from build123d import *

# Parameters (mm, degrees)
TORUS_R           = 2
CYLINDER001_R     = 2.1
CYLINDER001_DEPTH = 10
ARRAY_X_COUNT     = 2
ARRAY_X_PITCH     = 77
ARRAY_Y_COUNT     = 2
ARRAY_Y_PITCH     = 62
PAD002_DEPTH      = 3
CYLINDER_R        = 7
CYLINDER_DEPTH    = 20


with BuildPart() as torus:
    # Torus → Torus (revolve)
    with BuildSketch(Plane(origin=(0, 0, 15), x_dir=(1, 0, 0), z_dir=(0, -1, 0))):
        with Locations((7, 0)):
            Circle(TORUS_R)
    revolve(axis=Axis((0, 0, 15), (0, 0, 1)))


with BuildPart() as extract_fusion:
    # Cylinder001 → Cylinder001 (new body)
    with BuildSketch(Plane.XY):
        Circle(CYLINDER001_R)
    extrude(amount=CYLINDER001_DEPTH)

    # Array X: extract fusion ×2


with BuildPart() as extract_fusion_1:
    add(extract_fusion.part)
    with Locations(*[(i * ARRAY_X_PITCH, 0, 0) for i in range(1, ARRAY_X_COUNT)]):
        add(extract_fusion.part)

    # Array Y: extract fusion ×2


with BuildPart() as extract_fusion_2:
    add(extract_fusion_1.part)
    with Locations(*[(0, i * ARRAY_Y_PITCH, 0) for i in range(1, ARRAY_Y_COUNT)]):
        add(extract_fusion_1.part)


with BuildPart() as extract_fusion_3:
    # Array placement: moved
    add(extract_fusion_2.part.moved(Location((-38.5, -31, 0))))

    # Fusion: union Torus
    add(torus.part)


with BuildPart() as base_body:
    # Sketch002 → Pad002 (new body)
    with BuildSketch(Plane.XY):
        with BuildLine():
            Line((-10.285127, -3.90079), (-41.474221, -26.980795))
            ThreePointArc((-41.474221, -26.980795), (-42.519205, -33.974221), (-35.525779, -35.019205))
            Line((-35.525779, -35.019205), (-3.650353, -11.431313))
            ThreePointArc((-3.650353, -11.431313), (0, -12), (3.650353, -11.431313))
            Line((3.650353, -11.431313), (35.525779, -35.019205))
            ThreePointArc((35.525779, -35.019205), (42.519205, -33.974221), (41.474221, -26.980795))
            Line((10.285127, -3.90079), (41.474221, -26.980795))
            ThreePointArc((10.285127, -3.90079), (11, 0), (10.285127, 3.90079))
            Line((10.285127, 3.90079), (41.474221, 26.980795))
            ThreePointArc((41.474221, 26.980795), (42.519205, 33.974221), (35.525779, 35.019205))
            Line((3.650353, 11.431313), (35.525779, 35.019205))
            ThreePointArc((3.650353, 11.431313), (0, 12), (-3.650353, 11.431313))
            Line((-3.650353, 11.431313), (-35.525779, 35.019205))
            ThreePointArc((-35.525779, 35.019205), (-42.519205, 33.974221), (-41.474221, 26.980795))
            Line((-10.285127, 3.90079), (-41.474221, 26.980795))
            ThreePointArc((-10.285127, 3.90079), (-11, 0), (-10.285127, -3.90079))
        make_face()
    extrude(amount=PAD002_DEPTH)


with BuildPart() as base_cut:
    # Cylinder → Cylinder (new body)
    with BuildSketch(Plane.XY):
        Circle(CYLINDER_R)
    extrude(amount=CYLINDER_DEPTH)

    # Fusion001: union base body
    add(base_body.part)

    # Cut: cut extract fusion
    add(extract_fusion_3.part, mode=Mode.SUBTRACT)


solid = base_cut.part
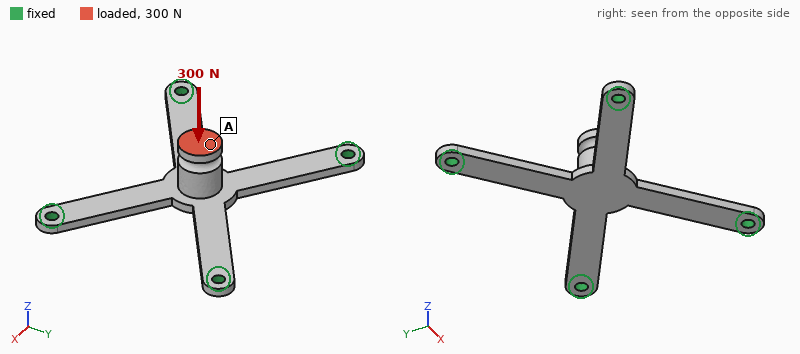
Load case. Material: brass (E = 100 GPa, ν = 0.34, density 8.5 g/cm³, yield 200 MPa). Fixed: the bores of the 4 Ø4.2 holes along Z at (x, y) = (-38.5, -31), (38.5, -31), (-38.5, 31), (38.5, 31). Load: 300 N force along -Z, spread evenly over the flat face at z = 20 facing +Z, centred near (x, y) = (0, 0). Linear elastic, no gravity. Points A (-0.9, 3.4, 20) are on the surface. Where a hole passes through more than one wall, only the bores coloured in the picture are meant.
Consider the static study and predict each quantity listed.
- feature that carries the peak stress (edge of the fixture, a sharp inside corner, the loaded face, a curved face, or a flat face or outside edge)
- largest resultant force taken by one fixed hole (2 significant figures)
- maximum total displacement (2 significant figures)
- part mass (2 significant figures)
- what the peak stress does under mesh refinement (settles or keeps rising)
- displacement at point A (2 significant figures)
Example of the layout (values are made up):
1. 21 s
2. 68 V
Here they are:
1. edge of the fixture
2. 77 N
3. 0.20 mm
4. 73 g
5. keeps rising
6. 0.20 mm
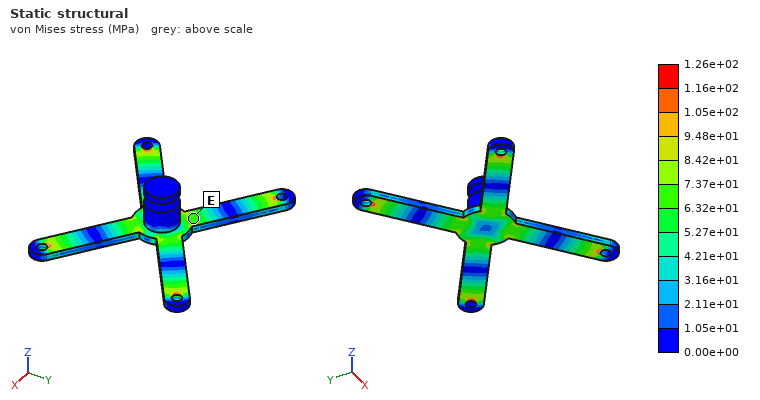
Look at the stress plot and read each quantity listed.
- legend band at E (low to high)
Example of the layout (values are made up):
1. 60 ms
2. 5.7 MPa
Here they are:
1. 6.32e+01 to 7.37e+01 MPa
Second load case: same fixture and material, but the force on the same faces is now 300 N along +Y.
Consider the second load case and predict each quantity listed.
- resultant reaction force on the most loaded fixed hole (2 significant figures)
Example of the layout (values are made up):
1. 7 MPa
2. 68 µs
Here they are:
1. 130 N
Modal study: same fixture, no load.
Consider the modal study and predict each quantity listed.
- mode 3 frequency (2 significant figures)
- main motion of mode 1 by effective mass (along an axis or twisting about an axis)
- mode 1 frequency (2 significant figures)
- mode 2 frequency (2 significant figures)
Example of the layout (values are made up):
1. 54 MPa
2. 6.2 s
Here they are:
1. 2300 Hz
2. along Z
3. 950 Hz
4. 2000 Hz
